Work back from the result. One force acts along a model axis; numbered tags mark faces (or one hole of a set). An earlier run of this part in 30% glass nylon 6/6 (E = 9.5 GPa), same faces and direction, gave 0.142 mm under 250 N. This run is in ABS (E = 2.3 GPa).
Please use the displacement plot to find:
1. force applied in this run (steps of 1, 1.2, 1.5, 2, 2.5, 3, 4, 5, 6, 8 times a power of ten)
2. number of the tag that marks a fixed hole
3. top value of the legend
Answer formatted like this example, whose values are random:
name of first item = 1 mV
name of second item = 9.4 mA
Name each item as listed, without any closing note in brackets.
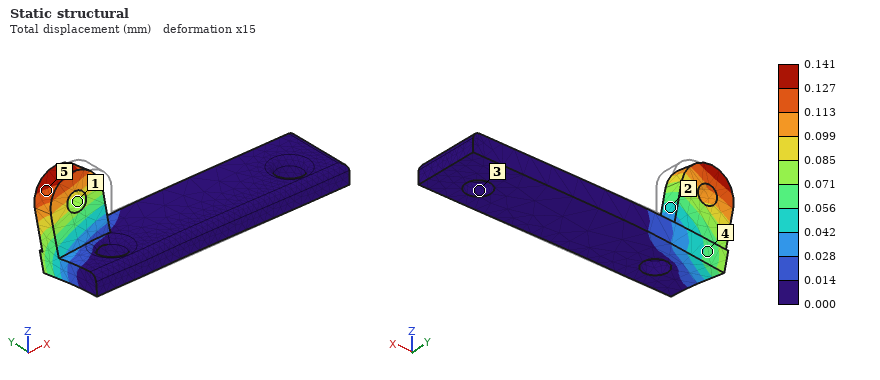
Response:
force applied in this run = 60 N
number of the tag that marks a fixed hole = 3
top value of the legend = 0.141 mm
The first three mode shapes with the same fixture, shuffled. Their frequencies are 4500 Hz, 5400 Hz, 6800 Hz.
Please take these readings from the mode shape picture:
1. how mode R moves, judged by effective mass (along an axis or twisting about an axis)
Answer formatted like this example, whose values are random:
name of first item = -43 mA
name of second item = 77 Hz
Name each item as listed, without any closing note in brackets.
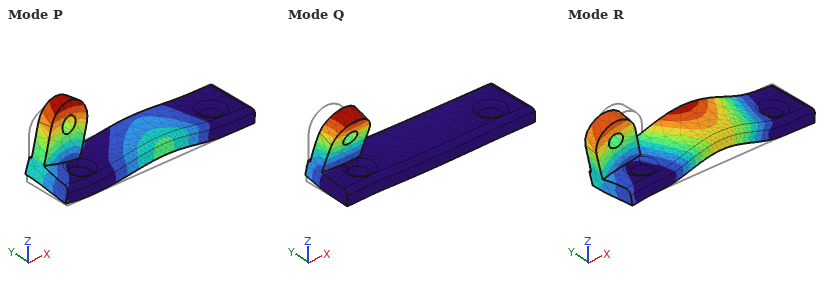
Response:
how mode R moves, judged by effective mass = along Z
